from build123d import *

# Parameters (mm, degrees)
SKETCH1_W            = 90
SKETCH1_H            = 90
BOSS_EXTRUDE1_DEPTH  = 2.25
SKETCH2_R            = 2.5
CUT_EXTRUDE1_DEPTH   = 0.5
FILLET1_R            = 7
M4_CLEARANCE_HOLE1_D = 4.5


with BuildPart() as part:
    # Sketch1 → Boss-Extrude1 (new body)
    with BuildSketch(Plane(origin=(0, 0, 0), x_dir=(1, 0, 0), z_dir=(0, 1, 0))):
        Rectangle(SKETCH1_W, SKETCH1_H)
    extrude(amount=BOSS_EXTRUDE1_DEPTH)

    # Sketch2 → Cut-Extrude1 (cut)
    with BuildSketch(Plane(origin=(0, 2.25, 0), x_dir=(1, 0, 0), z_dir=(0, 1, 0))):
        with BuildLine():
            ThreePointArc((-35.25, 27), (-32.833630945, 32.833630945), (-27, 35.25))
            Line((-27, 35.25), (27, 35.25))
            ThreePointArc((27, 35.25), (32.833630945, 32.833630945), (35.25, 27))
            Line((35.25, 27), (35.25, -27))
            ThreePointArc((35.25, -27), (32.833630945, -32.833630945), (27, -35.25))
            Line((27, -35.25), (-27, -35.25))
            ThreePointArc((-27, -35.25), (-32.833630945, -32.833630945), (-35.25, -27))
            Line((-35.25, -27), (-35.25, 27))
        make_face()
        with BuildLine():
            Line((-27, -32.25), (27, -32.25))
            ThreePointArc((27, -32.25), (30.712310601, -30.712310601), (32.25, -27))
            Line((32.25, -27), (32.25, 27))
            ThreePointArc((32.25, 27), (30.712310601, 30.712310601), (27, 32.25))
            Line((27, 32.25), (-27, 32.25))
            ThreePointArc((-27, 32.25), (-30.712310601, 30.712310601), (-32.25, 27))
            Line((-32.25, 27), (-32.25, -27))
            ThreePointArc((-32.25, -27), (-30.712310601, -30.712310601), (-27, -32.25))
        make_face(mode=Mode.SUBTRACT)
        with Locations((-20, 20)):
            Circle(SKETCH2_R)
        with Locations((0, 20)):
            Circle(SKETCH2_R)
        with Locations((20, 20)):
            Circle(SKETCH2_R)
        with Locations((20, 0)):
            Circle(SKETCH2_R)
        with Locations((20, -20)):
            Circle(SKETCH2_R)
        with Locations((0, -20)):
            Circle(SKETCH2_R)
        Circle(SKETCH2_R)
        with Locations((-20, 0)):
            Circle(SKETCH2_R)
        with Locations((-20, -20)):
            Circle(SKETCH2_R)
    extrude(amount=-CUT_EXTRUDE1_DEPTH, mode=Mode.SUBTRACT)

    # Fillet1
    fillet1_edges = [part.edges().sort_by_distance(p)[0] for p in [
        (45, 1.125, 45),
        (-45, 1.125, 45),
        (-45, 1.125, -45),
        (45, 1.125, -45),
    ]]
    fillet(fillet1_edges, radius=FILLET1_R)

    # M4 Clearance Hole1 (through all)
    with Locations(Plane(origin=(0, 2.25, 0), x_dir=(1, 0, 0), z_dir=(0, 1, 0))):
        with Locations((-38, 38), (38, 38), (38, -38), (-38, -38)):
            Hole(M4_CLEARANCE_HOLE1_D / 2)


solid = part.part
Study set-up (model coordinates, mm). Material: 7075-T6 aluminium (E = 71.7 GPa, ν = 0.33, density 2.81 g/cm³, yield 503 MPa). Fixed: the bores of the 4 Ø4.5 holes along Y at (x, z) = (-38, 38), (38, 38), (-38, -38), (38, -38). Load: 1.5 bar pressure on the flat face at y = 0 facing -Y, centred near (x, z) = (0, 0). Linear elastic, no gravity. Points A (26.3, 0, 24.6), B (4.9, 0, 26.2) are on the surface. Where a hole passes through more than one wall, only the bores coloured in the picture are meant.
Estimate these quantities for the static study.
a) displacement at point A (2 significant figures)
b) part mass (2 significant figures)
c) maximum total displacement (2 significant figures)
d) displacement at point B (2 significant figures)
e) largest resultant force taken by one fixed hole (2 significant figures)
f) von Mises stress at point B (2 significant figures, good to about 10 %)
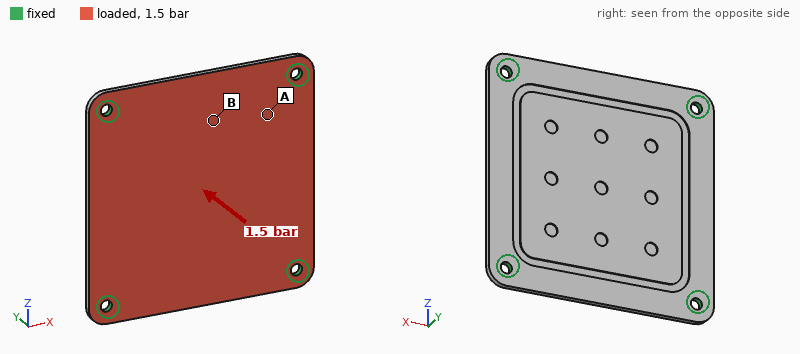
0.20 mm
49 g
0.51 mm
0.36 mm
300 N
49 MPa
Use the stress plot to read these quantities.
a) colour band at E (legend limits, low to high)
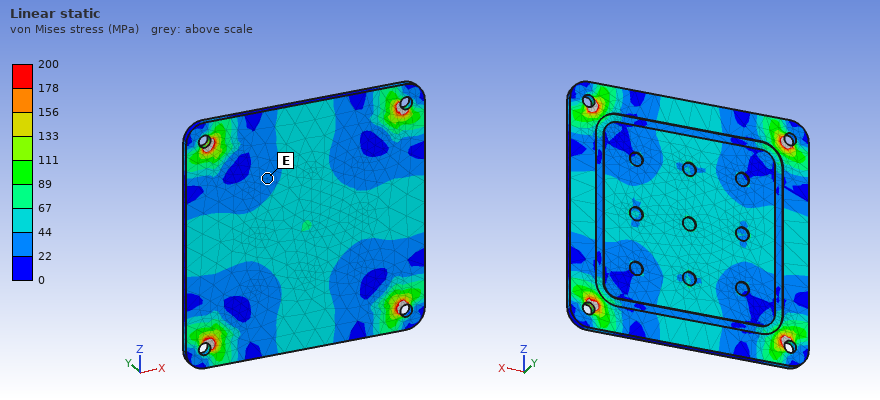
22 to 44 MPa
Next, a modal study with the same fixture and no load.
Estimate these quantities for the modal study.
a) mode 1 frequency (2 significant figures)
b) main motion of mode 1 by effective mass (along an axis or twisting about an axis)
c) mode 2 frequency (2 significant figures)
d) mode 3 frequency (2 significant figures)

1300 Hz
along Y
2300 Hz
2300 Hz
